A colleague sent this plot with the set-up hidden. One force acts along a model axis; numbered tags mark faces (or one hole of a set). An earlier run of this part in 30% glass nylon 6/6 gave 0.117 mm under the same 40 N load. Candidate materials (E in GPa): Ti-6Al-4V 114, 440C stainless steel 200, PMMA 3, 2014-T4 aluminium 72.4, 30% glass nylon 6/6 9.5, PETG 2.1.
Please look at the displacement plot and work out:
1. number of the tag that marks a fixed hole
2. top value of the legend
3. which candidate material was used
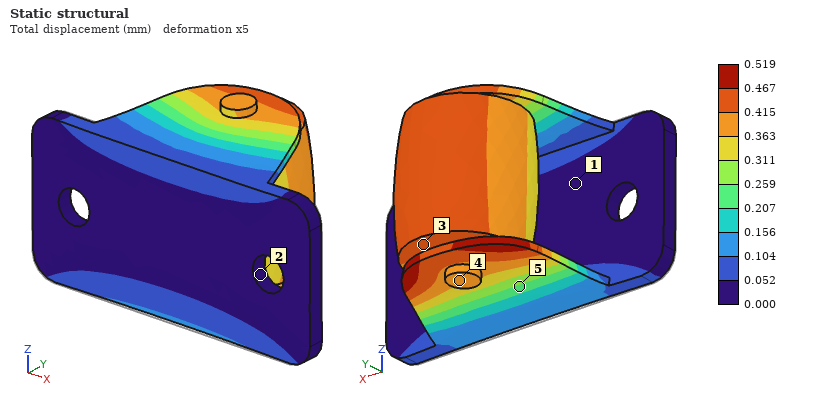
2
0.519 mm
PETG
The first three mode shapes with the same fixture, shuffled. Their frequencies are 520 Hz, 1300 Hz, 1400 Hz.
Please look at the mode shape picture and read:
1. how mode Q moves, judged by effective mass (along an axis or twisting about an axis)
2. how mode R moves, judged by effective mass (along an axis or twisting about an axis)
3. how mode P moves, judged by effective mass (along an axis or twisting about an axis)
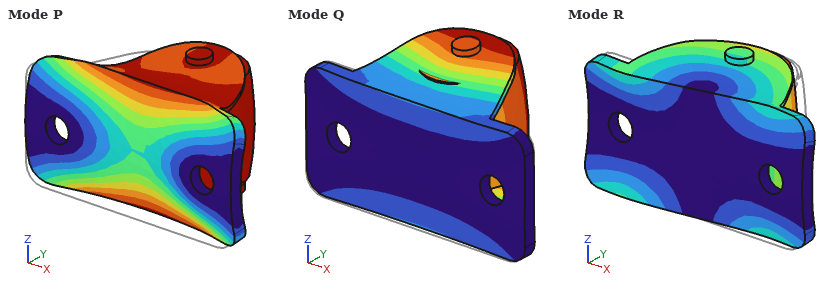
along Z
along X
along Y
